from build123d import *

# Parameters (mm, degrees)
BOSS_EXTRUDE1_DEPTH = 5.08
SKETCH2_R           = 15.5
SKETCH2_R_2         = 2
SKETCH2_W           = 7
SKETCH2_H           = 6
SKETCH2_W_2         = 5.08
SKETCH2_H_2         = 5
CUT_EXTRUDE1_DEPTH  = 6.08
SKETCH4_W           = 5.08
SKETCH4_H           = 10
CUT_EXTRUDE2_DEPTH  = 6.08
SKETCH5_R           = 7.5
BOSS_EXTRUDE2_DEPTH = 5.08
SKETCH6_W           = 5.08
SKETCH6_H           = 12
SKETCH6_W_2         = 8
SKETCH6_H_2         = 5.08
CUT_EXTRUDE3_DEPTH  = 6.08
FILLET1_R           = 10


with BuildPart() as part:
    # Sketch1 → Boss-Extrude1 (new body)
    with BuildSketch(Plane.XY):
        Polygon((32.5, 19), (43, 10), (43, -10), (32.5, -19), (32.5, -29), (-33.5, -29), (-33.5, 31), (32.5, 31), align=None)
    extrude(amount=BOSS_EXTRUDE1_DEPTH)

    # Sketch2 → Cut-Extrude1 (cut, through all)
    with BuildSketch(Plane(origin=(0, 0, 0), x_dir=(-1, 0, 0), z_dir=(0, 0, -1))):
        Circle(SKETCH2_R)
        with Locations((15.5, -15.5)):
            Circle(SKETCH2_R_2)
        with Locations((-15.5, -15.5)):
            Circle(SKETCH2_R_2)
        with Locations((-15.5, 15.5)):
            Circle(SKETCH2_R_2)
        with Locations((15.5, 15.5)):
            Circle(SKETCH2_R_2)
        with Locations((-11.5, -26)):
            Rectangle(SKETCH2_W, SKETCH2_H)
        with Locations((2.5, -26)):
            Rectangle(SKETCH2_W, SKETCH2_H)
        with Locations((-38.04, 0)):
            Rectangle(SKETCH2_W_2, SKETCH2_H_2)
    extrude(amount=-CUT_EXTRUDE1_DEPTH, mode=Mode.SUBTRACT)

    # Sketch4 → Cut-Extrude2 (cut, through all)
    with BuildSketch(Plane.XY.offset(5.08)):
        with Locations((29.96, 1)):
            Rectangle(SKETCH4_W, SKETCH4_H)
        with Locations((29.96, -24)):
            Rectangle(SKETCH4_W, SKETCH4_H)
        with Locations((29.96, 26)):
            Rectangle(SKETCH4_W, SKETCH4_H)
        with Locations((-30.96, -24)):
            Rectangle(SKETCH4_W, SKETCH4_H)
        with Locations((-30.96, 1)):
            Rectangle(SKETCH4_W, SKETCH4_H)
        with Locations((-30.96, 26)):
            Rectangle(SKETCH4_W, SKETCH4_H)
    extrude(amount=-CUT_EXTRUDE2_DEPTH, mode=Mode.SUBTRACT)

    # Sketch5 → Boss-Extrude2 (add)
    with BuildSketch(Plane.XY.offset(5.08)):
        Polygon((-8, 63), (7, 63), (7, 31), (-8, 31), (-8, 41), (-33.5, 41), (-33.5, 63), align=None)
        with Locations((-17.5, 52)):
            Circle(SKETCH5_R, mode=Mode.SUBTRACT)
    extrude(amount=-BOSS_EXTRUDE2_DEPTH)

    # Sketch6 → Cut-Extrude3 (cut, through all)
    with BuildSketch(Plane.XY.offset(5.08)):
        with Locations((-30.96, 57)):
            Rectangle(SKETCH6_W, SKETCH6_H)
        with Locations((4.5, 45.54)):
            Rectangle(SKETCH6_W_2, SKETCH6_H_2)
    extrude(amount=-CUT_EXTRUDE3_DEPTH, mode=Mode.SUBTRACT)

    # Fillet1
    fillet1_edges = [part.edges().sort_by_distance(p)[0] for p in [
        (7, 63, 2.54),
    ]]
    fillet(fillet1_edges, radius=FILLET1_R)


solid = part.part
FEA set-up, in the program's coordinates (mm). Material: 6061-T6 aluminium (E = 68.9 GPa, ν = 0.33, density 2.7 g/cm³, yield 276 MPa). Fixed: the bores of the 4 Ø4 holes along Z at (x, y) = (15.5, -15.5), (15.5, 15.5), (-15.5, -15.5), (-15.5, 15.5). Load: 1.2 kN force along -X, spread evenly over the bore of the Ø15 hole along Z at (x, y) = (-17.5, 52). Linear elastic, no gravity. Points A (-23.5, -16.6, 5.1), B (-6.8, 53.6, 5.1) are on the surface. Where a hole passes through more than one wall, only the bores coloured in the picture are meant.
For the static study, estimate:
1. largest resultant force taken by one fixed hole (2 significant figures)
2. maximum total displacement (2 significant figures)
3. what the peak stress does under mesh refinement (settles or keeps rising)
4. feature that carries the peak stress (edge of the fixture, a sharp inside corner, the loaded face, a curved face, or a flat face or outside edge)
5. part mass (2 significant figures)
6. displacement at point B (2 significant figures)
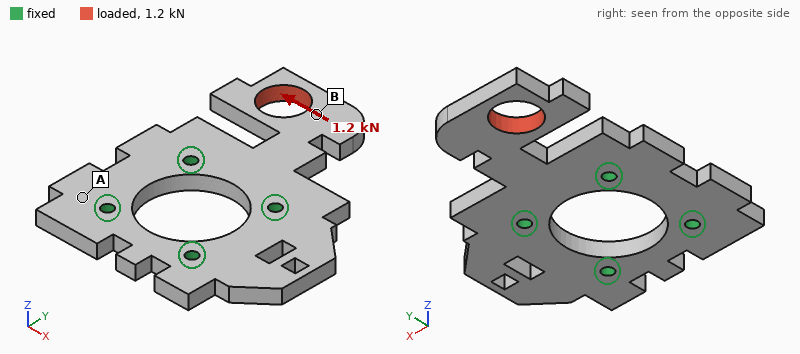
1.4 kN
0.29 mm
keeps rising
a sharp inside corner
52 g
0.14 mm
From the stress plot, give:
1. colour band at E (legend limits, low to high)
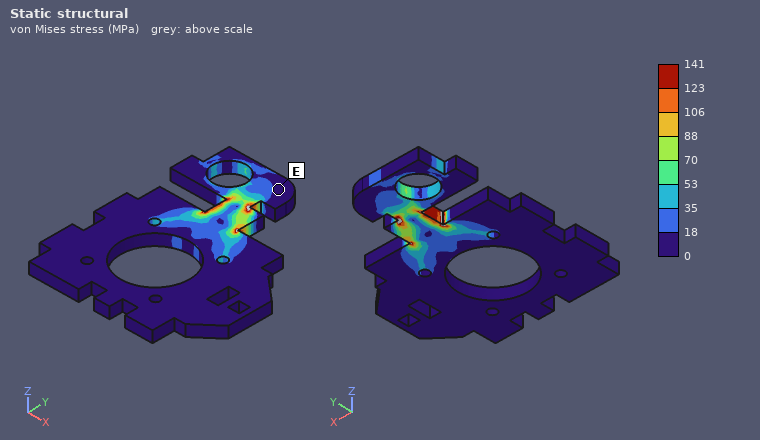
0 to 18 MPa
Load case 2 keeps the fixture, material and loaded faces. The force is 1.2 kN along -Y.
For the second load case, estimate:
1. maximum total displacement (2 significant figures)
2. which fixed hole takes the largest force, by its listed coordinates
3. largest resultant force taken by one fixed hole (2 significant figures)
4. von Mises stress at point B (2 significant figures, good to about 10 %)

0.35 mm
(-15.5, 15.5)
1.4 kN
21 MPa
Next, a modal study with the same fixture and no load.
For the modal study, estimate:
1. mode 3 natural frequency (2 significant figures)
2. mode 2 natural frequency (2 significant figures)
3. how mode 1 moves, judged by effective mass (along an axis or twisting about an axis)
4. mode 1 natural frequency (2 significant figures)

3700 Hz
3100 Hz
along Z
1500 Hz
